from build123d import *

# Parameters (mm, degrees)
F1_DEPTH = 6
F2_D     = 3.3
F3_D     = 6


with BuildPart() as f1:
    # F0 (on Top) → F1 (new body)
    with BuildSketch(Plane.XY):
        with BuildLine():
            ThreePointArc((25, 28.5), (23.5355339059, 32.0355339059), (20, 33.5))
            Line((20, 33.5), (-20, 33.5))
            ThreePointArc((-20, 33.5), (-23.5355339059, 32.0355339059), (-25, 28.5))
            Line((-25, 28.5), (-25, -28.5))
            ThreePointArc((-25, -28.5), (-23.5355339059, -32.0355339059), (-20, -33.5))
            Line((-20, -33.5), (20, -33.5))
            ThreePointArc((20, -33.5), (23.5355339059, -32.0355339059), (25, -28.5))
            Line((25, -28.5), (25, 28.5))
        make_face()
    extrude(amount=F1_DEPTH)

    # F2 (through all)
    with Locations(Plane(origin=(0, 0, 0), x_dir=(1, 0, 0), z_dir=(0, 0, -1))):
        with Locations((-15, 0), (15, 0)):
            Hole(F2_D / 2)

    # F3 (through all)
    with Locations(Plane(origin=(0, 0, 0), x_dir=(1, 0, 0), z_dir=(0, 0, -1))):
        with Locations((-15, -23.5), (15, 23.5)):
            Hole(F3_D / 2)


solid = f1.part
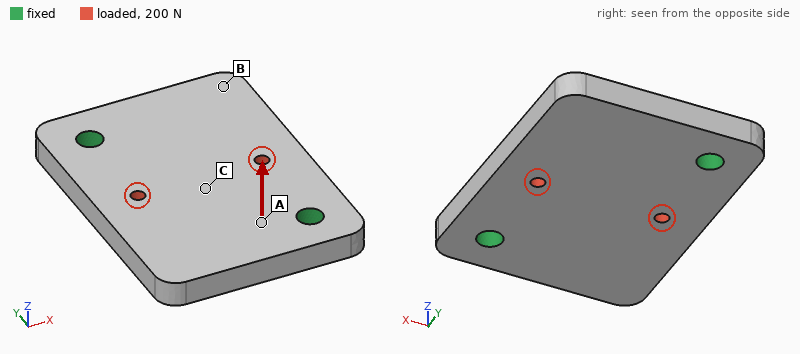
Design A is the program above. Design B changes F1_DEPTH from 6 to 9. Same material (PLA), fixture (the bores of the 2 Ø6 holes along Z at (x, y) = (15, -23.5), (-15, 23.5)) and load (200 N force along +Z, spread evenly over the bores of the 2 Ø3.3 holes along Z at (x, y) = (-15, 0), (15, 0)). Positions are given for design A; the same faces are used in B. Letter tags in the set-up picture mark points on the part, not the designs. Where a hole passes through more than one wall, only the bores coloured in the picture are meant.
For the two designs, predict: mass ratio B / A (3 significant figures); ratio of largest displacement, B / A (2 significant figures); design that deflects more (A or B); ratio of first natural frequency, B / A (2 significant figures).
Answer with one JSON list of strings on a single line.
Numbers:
["1.50", "0.34", "A", "1.4"]
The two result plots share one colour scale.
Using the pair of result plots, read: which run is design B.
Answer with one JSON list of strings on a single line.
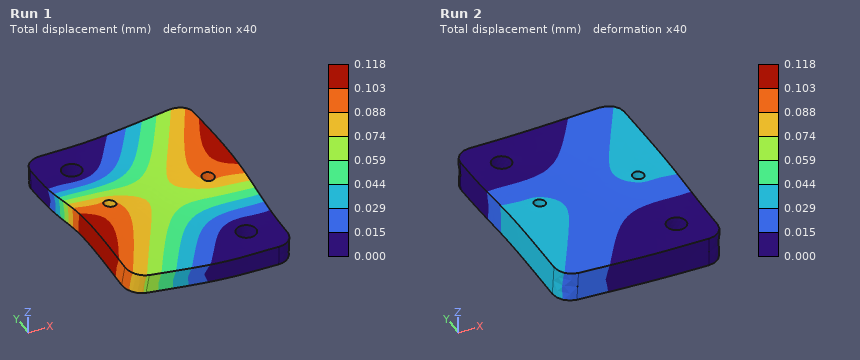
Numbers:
["Run 2"]
